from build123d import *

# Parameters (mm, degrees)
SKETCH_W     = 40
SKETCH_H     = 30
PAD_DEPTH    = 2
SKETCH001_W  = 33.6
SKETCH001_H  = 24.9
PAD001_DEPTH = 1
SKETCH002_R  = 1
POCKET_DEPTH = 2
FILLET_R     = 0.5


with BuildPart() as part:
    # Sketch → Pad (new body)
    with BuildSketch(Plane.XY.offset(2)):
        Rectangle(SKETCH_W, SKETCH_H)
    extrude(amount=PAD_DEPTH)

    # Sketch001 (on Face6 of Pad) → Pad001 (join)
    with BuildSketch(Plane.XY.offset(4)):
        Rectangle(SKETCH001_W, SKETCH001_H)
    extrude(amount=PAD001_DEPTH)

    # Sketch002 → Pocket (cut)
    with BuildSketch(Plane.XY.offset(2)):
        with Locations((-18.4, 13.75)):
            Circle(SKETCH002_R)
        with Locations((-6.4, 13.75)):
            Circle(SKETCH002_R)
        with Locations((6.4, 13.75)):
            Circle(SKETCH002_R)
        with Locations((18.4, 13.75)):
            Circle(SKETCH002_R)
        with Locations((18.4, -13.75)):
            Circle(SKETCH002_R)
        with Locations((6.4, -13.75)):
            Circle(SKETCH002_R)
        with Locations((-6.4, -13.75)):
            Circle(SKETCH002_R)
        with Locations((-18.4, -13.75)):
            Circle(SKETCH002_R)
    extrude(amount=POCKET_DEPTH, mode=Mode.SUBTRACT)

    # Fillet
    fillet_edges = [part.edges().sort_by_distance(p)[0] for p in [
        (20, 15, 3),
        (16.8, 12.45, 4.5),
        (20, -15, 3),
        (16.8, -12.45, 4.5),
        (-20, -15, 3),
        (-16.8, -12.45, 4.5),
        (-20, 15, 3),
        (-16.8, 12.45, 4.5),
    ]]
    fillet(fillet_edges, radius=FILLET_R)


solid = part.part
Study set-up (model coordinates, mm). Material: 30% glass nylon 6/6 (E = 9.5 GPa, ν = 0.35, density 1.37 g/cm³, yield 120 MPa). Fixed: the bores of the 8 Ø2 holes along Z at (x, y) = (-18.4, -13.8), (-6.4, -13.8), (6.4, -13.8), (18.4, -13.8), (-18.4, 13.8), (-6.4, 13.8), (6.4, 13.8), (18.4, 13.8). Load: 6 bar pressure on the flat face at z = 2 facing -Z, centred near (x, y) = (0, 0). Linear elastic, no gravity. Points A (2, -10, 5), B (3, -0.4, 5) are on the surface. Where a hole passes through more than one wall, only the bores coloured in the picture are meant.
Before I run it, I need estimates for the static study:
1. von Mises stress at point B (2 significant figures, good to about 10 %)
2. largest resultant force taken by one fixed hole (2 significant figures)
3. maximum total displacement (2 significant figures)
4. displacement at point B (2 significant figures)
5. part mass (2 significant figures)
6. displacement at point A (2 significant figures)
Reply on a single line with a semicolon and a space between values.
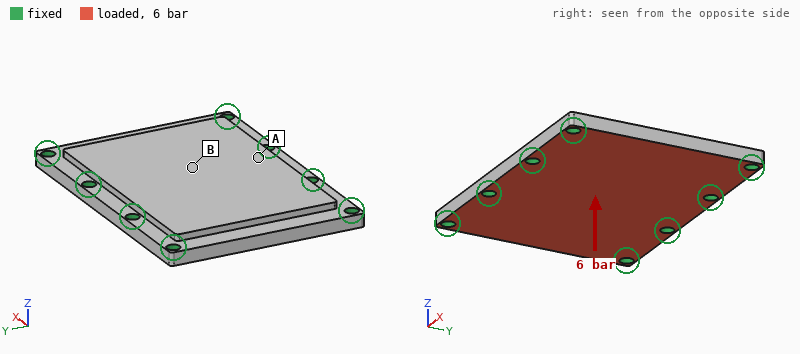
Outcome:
19 MPa; 130 N; 0.11 mm; 0.082 mm; 4.4 g; 0.034 mm
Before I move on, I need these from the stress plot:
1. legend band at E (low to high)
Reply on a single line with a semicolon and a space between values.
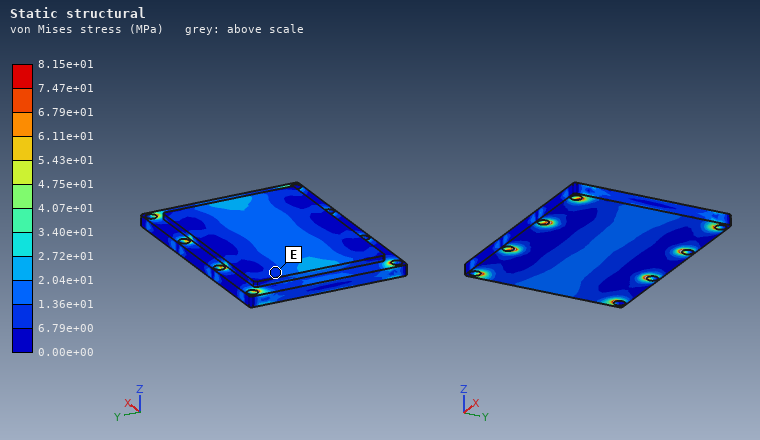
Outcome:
6.79e+00 to 1.36e+01 MPa
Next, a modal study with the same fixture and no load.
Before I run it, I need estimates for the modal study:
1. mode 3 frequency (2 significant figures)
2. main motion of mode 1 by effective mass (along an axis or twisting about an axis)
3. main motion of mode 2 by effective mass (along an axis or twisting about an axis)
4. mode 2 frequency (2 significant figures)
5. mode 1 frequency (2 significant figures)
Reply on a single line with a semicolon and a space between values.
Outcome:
13 kHz; along Z; twisting about Y; 8600 Hz; 7500 Hz
